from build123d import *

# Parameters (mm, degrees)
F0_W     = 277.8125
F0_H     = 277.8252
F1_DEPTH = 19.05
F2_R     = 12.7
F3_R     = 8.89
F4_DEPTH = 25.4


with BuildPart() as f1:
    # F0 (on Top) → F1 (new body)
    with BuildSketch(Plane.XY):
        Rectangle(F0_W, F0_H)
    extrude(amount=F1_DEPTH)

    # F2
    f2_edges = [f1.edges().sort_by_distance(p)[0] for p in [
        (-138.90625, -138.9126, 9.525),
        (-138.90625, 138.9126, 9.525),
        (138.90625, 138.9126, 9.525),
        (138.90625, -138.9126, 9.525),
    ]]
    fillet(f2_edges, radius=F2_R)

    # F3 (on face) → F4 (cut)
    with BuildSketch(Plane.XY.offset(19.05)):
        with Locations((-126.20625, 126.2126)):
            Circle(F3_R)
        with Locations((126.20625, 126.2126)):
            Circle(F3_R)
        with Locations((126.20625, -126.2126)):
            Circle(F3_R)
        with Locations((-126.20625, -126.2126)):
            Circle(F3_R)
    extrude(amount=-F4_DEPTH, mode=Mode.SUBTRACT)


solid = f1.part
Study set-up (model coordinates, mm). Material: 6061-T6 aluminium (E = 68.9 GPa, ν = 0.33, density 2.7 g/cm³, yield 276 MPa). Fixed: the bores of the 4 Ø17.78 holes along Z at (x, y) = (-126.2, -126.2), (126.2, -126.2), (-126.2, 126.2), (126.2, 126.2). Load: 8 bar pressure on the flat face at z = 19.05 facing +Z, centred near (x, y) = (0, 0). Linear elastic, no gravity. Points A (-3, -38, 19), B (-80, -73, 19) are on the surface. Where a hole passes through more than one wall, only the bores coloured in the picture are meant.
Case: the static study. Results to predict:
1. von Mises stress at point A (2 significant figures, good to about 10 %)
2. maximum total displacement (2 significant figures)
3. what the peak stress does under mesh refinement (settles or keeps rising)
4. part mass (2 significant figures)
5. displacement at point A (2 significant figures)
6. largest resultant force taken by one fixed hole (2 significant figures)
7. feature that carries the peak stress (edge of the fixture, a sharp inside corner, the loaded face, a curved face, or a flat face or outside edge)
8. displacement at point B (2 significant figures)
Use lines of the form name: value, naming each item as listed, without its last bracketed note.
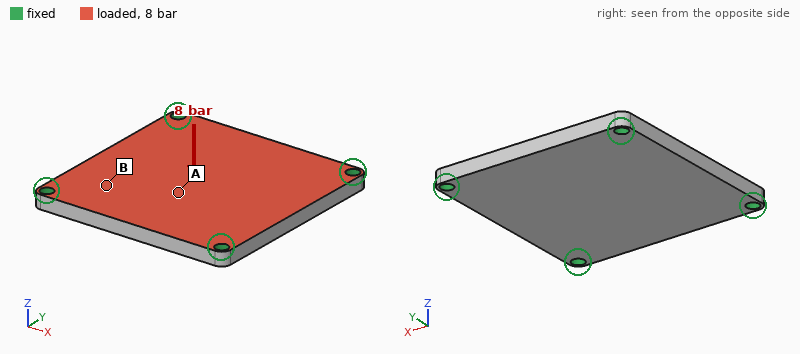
von Mises stress at point A: 46 MPa
maximum total displacement: 0.62 mm
what the peak stress does under mesh refinement: keeps rising
part mass: 3.9 kg
displacement at point A: 0.58 mm
largest resultant force taken by one fixed hole: 15 kN
feature that carries the peak stress: edge of the fixture
displacement at point B: 0.32 mm
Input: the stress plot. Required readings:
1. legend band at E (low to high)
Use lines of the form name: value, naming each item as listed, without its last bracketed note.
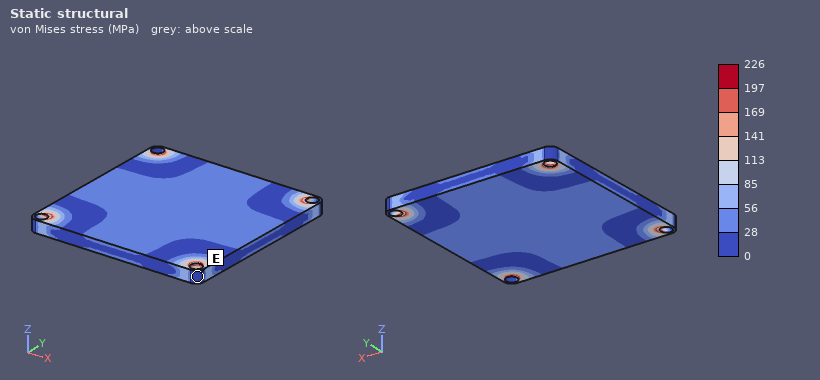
legend band at E: 0 to 28 MPa
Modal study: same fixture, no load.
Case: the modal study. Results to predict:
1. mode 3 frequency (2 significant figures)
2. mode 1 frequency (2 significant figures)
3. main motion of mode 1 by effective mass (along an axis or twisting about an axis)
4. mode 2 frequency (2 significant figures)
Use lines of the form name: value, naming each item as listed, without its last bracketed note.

mode 3 frequency: 1700 Hz
mode 1 frequency: 960 Hz
main motion of mode 1 by effective mass: along Z
mode 2 frequency: 1700 Hz
